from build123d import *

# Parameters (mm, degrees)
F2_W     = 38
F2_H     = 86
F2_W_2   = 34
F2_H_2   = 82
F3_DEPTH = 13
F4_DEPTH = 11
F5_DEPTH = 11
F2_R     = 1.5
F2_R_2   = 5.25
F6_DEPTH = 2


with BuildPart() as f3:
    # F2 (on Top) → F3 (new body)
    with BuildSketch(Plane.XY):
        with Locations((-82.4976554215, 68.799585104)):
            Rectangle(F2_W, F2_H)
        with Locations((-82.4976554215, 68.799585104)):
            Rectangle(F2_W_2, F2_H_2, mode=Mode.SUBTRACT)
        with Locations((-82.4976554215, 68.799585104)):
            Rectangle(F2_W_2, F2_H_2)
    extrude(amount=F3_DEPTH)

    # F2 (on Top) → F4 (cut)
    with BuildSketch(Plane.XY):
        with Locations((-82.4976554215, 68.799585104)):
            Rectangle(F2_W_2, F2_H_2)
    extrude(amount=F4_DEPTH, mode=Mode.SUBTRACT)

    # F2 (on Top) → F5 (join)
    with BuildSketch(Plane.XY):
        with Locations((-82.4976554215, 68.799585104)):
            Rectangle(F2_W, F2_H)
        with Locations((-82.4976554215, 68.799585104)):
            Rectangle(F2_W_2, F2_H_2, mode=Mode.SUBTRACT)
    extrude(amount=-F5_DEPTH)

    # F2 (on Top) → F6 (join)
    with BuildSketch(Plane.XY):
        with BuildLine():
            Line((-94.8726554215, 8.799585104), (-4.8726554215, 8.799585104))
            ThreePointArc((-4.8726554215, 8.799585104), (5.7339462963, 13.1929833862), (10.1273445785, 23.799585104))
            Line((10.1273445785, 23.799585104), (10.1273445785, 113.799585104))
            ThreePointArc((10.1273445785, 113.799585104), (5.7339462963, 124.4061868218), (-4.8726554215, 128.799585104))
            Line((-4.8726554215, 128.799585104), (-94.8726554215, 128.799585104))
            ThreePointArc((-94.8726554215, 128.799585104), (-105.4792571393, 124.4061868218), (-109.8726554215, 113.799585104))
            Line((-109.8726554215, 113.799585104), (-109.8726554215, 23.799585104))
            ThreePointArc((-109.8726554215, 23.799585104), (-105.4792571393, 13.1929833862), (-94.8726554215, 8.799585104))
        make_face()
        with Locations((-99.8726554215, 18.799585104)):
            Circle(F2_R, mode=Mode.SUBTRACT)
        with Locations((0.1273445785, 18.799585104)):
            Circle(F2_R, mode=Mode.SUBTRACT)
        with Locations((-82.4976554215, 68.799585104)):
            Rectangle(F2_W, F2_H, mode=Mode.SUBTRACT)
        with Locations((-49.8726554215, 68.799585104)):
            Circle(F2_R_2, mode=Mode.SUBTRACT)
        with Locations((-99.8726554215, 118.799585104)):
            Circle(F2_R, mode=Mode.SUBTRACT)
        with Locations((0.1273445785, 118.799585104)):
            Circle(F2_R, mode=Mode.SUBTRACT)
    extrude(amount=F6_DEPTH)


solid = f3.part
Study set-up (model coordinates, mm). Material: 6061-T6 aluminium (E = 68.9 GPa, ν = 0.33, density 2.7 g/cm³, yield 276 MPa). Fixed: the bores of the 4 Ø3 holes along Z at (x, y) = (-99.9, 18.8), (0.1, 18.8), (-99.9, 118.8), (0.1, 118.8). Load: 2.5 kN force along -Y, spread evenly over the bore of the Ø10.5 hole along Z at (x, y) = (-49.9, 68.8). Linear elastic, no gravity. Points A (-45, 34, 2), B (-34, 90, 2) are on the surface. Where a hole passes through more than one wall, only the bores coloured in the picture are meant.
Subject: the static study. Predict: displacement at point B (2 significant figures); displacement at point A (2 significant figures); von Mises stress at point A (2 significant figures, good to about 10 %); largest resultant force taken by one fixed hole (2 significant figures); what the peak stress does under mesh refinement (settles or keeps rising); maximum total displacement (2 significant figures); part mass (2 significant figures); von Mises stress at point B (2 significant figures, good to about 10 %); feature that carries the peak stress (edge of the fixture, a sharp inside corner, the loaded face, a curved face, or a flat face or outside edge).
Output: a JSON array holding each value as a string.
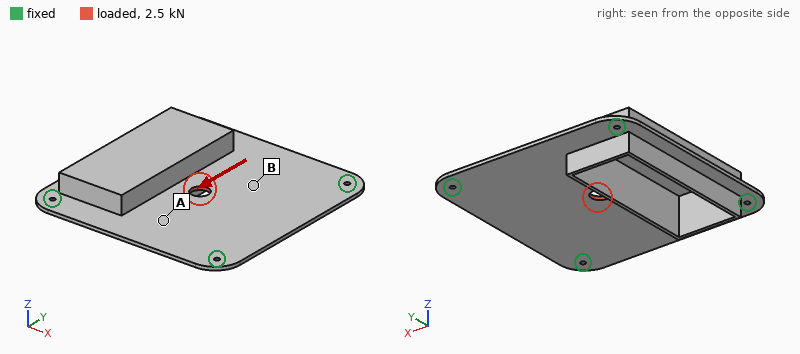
["30 µm", "51 µm", "6.0 MPa", "1.2 kN", "keeps rising", "81 µm", "100 g", "15 MPa", "edge of the fixture"]
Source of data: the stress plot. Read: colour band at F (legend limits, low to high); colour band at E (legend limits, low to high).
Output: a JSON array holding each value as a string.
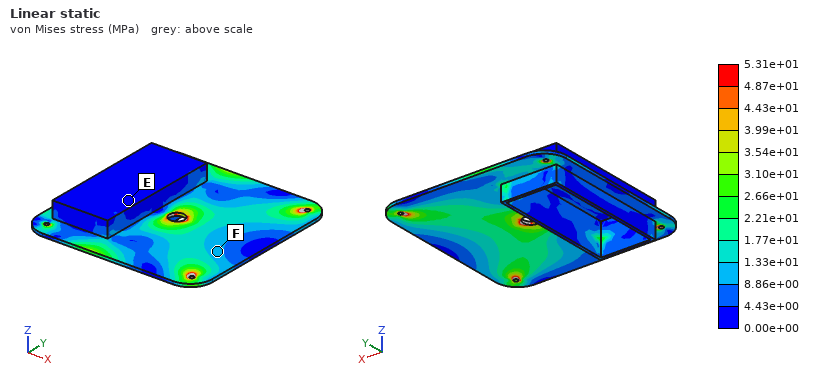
["8.86e+00 to 1.33e+01 MPa", "0.00e+00 to 4.43e+00 MPa"]
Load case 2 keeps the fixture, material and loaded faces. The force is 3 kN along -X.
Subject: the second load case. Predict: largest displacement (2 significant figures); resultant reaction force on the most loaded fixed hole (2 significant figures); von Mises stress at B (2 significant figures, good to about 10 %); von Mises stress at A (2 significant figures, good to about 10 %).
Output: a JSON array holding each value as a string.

["57 µm", "1.1 kN", "24 MPa", "17 MPa"]
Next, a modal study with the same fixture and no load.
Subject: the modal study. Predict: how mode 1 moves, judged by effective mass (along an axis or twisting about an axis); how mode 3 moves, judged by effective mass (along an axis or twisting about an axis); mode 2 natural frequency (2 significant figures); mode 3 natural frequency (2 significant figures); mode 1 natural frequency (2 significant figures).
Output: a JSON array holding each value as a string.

["along Z", "twisting about X", "1200 Hz", "1900 Hz", "700 Hz"]
